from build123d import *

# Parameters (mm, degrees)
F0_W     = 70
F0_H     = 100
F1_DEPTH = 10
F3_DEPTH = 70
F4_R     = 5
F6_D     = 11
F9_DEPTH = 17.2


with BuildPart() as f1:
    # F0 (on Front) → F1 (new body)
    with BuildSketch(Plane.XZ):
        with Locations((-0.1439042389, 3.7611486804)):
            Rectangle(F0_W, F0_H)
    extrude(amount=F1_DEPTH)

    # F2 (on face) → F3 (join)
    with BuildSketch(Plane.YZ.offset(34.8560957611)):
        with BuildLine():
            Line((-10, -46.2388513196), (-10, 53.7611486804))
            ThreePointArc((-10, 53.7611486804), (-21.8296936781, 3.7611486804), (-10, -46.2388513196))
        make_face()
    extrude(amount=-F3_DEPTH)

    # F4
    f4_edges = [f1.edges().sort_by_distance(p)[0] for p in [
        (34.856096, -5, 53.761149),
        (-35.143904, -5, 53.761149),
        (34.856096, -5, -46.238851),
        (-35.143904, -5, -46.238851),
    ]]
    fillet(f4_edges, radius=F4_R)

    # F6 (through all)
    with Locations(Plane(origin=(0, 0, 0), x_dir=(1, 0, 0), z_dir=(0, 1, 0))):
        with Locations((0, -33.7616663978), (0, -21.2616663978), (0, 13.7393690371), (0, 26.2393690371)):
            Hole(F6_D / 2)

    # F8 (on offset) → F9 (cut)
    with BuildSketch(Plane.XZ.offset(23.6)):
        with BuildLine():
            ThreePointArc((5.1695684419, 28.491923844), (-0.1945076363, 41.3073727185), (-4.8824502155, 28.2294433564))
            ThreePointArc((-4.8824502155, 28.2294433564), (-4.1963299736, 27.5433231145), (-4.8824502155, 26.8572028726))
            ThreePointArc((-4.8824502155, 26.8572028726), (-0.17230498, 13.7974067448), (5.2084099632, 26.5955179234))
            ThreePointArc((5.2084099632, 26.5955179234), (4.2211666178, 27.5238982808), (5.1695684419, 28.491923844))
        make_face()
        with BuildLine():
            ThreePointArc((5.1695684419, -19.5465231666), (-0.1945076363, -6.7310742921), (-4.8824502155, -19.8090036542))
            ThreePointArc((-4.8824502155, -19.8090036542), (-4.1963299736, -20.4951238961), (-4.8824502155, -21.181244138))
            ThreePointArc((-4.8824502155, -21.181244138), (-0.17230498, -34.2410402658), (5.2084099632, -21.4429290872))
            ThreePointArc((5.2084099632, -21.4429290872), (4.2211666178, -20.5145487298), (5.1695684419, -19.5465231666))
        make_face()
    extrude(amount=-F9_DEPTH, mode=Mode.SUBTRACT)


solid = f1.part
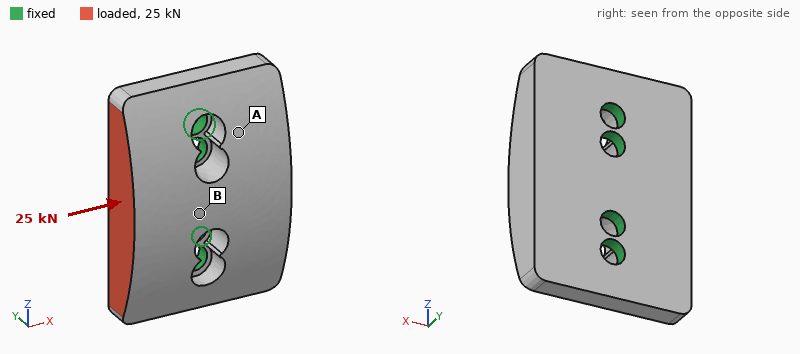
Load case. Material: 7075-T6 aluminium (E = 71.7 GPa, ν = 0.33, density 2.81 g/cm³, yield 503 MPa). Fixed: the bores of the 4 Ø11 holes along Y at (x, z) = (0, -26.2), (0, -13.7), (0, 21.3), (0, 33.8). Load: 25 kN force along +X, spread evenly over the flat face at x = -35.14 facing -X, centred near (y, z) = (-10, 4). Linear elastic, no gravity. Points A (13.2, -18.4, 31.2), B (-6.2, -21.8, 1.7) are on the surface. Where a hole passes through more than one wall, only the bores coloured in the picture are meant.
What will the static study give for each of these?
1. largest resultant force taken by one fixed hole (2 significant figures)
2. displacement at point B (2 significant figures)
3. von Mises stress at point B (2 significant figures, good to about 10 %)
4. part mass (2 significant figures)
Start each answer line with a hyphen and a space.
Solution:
- 6.7 kN
- 37 µm
- 29 MPa
- 320 g
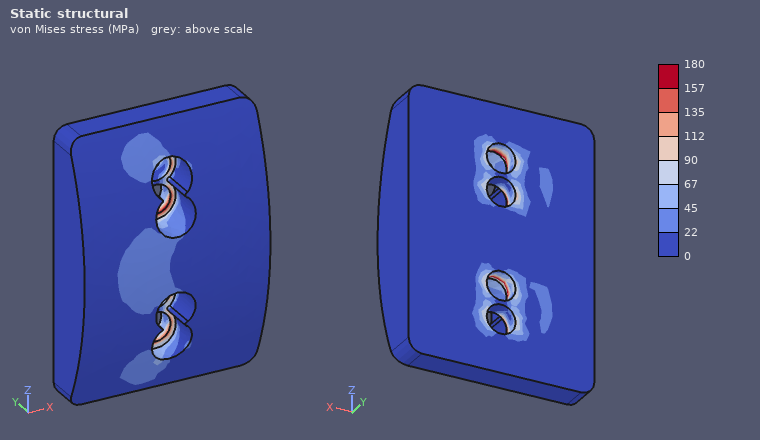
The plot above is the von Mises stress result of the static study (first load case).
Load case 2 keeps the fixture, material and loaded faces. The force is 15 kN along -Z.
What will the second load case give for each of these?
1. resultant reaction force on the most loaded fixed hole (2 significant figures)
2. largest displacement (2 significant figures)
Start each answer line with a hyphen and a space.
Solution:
- 7.1 kN
- 31 µm
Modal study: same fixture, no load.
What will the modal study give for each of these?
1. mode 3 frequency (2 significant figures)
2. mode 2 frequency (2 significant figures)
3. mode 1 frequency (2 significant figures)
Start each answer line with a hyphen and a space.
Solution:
- 9000 Hz
- 8900 Hz
- 4200 Hz
